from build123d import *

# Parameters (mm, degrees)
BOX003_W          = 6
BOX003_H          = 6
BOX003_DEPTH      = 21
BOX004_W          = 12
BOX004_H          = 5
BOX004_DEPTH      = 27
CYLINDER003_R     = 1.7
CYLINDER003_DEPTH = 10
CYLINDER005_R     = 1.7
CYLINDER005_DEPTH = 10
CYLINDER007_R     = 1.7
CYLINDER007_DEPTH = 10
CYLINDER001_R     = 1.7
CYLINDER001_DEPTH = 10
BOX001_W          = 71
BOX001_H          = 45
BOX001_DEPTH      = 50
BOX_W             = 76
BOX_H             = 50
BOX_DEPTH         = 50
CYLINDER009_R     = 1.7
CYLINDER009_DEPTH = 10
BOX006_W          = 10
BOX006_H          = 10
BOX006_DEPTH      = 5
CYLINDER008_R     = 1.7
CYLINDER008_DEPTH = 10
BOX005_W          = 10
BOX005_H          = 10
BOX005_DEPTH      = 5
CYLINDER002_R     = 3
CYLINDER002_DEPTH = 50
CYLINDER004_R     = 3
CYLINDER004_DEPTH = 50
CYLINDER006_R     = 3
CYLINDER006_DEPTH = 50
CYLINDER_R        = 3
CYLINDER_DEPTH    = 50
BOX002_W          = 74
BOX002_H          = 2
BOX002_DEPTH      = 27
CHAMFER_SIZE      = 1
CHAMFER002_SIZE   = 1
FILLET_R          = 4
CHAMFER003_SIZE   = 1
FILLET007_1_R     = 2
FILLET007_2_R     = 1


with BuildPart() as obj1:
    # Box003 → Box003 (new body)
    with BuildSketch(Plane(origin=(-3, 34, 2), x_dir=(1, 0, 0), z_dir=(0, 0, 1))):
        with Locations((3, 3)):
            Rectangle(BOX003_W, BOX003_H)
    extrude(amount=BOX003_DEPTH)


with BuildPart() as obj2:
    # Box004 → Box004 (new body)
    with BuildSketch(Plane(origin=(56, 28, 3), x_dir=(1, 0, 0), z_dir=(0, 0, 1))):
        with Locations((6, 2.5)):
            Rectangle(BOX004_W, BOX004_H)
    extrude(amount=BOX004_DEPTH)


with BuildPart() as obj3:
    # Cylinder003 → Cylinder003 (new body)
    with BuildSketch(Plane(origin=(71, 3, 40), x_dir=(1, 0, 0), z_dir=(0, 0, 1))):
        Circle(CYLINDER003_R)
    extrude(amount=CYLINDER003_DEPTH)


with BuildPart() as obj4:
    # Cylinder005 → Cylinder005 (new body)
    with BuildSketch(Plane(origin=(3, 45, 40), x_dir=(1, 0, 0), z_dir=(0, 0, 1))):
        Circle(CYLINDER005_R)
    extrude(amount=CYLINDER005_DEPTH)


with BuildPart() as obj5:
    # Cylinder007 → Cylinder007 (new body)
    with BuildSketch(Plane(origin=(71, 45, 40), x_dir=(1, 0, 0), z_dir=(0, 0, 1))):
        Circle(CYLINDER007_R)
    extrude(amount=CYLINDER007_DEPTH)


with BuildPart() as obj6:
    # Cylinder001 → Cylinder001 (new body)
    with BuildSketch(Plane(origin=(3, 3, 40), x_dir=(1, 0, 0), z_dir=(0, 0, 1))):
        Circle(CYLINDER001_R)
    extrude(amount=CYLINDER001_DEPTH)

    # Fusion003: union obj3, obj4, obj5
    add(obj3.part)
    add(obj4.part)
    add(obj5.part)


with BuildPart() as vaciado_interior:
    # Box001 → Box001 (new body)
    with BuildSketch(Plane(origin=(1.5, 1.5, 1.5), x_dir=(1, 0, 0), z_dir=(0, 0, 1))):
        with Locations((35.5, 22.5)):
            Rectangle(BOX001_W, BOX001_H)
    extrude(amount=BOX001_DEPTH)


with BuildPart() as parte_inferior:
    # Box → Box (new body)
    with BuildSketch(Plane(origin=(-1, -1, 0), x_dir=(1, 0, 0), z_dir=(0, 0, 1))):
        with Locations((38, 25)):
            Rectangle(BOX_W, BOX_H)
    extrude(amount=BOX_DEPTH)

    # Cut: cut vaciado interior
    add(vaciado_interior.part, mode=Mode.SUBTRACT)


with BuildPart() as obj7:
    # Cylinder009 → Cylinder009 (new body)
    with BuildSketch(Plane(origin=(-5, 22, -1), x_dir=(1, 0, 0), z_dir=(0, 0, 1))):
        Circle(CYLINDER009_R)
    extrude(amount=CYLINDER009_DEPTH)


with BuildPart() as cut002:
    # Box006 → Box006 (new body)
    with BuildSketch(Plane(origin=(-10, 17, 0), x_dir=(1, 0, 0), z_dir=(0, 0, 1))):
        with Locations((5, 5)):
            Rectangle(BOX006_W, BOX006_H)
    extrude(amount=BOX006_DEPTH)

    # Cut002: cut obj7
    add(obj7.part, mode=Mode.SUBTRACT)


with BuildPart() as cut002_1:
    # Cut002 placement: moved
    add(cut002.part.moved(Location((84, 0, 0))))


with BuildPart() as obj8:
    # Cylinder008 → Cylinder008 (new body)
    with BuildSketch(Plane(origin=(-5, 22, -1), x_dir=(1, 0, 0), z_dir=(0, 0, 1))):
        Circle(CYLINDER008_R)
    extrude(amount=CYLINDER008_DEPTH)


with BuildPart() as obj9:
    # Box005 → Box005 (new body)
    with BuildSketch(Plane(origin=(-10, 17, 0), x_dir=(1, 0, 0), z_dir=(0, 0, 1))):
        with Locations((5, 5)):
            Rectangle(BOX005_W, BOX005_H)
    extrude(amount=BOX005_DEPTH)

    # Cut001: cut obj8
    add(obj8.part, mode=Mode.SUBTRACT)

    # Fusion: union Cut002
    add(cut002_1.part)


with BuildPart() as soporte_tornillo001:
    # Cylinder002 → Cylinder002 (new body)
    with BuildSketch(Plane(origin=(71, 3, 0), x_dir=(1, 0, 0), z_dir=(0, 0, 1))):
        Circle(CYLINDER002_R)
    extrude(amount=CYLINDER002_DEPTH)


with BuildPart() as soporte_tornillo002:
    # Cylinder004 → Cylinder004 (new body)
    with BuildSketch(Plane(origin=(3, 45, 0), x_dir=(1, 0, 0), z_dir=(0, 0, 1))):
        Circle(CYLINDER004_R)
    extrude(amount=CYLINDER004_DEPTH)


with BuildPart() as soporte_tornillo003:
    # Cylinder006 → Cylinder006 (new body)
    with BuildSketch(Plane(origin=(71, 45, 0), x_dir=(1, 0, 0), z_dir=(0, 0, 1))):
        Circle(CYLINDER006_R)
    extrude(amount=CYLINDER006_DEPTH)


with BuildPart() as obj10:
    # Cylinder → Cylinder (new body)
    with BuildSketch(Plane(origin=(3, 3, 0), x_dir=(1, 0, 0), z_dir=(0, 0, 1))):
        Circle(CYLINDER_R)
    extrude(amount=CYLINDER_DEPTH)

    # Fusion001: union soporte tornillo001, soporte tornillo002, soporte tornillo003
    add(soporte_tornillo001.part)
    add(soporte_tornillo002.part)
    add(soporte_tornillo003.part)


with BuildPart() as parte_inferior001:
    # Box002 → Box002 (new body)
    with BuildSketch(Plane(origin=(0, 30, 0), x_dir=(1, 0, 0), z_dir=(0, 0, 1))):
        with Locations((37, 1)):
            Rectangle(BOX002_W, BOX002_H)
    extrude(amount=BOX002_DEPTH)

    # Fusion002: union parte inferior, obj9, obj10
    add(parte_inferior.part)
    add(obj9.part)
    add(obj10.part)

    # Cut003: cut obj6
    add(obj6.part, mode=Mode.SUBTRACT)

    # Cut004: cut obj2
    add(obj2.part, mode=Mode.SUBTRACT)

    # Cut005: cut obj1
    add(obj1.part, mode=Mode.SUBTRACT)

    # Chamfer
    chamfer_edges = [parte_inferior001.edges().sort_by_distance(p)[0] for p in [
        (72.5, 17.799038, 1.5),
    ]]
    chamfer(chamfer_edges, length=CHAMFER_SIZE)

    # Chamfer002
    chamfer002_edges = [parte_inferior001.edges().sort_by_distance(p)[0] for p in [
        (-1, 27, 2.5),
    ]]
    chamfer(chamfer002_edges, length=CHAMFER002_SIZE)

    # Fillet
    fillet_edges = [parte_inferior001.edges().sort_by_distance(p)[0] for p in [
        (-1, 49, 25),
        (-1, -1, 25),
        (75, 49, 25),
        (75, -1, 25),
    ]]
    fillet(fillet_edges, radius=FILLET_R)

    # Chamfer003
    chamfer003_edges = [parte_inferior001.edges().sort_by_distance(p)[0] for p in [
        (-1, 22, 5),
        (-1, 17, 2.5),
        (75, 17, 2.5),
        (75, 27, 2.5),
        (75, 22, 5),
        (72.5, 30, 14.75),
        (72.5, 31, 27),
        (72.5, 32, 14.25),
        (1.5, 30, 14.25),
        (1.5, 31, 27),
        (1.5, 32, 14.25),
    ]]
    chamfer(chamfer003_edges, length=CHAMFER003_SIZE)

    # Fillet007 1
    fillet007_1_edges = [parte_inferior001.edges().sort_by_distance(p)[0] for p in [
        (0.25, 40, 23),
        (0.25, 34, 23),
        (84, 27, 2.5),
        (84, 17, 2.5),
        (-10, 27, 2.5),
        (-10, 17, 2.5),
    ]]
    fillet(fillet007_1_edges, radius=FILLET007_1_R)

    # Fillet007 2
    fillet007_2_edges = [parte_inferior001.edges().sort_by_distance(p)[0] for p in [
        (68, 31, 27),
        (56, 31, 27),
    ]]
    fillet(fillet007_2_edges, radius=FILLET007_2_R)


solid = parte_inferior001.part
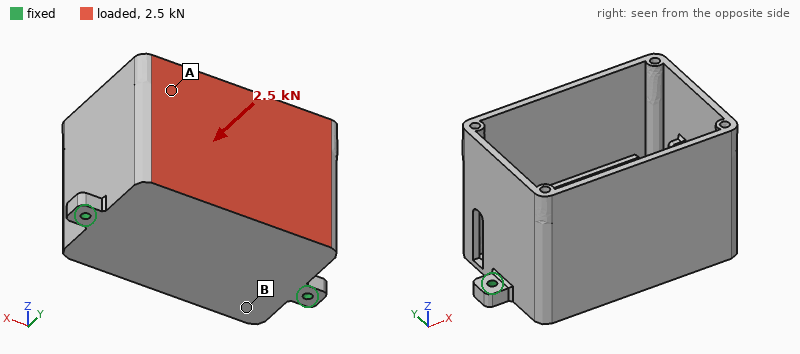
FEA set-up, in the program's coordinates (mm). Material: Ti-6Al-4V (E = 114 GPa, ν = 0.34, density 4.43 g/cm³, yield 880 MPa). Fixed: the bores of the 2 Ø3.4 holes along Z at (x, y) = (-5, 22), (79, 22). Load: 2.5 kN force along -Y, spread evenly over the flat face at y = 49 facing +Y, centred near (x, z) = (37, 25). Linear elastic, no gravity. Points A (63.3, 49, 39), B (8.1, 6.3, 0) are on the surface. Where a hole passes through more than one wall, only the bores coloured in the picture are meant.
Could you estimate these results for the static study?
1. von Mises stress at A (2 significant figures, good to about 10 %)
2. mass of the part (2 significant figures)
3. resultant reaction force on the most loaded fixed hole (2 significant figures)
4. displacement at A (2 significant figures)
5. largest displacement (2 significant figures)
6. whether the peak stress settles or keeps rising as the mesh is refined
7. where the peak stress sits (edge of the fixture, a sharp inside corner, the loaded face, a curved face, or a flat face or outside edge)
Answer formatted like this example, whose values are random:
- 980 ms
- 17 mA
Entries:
- 66 MPa
- 180 g
- 1.3 kN
- 0.53 mm
- 0.92 mm
- keeps rising
- edge of the fixture
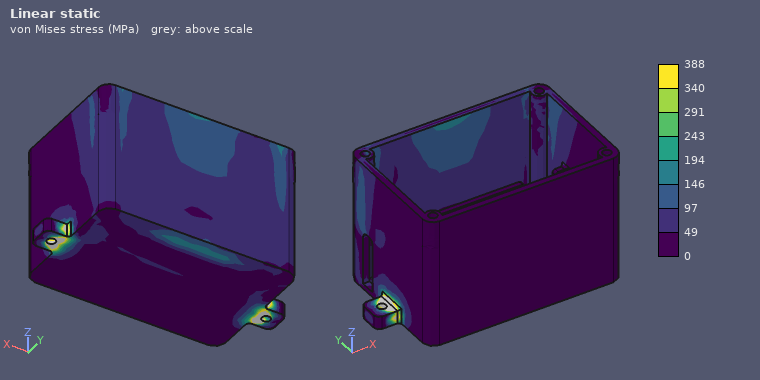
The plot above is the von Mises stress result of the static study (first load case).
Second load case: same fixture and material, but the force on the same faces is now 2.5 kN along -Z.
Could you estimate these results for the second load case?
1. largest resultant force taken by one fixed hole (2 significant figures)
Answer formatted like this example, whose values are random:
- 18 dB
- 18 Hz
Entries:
- 1.3 kN
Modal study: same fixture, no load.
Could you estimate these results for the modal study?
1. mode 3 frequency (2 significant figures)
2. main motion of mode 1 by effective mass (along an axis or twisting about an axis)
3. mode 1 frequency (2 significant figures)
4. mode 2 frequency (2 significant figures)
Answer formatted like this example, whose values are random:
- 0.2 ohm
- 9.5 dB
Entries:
- 2500 Hz
- along Y
- 920 Hz
- 1600 Hz
